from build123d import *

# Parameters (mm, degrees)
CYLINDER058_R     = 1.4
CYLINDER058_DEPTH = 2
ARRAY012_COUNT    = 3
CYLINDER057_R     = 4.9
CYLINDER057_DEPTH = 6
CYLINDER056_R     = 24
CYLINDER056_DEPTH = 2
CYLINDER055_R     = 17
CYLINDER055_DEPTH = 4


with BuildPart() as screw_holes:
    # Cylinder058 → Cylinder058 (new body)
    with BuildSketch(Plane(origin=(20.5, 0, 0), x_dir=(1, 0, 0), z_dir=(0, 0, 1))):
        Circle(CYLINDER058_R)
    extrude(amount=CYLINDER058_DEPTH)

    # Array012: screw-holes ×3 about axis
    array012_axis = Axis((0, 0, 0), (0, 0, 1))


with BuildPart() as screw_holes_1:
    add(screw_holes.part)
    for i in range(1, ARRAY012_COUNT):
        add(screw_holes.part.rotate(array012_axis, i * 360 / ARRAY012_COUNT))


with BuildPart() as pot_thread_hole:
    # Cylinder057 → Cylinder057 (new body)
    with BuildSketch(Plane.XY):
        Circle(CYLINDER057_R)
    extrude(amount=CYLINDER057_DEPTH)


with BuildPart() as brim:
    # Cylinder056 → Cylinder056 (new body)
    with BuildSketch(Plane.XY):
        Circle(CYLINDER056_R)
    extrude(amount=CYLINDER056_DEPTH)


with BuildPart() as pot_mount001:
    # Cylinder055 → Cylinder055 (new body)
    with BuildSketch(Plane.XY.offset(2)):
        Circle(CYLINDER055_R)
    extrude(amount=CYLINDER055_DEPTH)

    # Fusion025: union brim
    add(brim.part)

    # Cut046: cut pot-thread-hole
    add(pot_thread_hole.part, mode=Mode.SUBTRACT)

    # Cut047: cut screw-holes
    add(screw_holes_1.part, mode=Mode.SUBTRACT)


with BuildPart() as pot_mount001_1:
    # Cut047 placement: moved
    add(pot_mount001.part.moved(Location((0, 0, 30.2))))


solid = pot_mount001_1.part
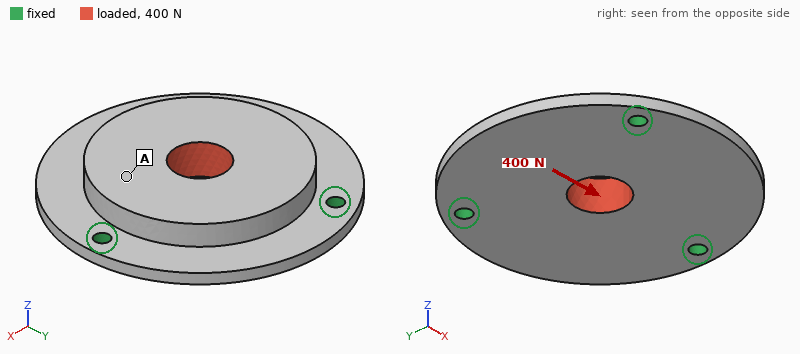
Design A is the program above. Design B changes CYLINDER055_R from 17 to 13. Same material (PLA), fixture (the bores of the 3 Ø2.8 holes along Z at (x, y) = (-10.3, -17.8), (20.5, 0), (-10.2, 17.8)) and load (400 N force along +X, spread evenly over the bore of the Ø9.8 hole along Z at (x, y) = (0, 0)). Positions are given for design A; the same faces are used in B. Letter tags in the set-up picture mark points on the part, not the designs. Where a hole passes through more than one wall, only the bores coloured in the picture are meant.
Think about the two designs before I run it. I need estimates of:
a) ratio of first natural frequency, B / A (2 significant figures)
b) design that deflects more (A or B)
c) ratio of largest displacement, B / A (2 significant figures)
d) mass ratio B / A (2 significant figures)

0.75
B
2.4
0.78
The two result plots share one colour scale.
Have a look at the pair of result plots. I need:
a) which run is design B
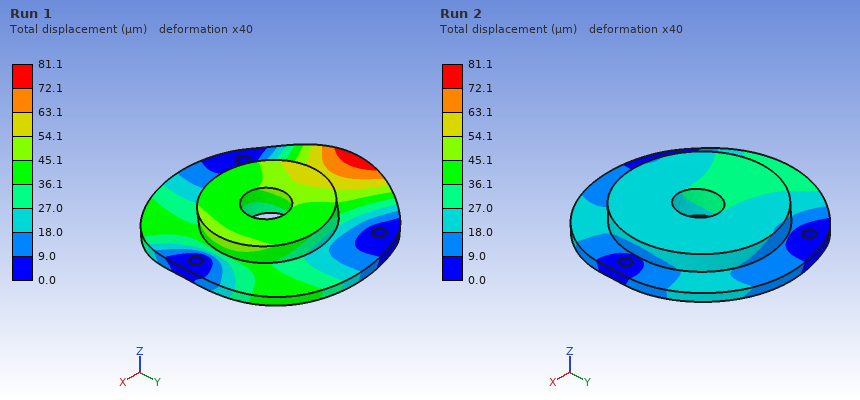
Run 1
